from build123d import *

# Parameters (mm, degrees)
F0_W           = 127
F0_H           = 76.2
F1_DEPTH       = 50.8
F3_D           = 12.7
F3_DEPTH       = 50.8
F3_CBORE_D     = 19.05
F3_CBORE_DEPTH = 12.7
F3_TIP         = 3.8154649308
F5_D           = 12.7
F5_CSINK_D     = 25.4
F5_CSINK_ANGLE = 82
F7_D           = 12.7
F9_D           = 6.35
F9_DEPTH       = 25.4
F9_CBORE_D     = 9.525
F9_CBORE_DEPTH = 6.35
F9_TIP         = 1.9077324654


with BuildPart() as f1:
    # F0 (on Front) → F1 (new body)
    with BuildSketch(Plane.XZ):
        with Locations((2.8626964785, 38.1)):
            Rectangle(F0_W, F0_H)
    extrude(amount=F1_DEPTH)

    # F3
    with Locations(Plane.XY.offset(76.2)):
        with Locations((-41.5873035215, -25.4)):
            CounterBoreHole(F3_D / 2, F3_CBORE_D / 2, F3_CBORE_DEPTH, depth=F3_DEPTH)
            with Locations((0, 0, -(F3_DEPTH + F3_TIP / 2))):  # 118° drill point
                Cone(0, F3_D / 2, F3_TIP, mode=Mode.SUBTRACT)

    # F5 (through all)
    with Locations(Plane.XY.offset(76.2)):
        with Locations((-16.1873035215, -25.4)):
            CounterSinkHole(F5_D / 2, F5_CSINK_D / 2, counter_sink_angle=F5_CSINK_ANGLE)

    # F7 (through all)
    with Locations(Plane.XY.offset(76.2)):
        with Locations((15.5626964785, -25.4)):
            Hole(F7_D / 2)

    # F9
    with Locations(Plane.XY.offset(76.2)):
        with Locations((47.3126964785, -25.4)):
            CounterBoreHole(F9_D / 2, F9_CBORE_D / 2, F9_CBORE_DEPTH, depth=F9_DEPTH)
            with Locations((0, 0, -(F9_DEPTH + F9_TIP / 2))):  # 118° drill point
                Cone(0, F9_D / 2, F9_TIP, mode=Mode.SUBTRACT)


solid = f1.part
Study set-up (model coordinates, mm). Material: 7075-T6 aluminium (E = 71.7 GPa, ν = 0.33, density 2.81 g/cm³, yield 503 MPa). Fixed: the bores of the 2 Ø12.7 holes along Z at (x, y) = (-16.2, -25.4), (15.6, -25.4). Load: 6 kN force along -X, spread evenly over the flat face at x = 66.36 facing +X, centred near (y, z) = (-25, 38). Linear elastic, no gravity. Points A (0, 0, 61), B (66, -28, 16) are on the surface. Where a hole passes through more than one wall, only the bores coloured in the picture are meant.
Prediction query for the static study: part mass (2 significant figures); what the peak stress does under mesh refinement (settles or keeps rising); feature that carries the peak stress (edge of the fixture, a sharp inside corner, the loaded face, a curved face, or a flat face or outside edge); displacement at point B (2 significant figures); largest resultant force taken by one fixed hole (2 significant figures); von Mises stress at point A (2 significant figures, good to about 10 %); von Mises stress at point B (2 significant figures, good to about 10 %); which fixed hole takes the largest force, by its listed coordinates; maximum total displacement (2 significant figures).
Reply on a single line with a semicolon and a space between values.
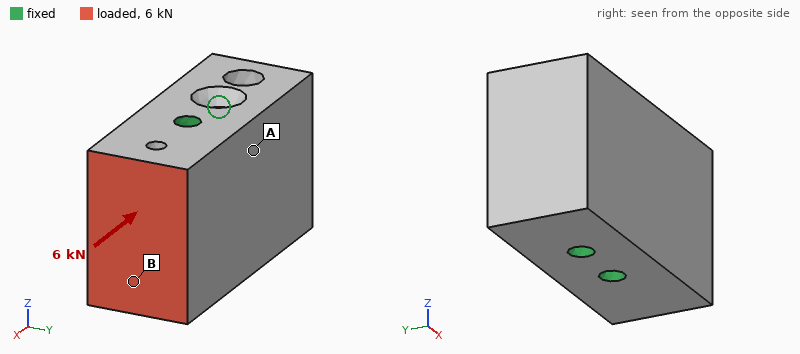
1.3 kg; keeps rising; a sharp inside corner; 1.2 µm; 4.9 kN; 0.57 MPa; 1.6 MPa; (15.6, -25.4); 1.4 µm
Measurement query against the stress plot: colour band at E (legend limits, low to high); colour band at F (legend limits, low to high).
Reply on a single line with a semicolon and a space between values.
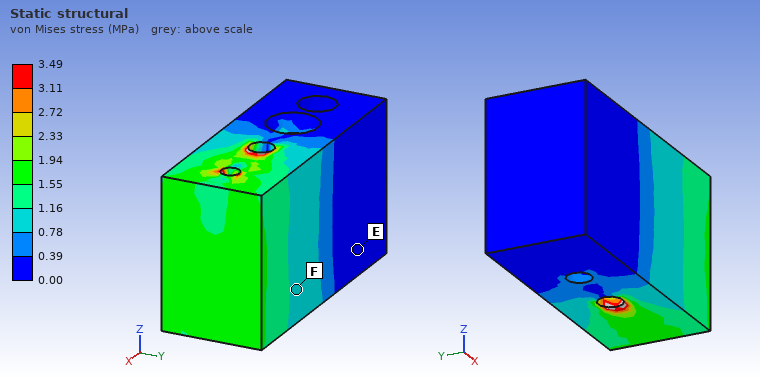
0.00 to 0.39 MPa; 0.78 to 1.16 MPa
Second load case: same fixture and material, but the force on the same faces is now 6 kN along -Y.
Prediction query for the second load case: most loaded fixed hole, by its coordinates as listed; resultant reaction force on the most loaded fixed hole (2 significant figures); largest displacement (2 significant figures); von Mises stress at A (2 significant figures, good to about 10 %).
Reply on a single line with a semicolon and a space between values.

(15.6, -25.4); 11 kN; 14 µm; 3.6 MPa
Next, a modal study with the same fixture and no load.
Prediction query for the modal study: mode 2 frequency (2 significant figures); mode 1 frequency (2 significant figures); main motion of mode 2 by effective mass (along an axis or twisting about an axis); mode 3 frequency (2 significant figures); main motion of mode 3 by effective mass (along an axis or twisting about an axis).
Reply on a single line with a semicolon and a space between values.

9800 Hz; 7700 Hz; along Y; 11 kHz; along Z
